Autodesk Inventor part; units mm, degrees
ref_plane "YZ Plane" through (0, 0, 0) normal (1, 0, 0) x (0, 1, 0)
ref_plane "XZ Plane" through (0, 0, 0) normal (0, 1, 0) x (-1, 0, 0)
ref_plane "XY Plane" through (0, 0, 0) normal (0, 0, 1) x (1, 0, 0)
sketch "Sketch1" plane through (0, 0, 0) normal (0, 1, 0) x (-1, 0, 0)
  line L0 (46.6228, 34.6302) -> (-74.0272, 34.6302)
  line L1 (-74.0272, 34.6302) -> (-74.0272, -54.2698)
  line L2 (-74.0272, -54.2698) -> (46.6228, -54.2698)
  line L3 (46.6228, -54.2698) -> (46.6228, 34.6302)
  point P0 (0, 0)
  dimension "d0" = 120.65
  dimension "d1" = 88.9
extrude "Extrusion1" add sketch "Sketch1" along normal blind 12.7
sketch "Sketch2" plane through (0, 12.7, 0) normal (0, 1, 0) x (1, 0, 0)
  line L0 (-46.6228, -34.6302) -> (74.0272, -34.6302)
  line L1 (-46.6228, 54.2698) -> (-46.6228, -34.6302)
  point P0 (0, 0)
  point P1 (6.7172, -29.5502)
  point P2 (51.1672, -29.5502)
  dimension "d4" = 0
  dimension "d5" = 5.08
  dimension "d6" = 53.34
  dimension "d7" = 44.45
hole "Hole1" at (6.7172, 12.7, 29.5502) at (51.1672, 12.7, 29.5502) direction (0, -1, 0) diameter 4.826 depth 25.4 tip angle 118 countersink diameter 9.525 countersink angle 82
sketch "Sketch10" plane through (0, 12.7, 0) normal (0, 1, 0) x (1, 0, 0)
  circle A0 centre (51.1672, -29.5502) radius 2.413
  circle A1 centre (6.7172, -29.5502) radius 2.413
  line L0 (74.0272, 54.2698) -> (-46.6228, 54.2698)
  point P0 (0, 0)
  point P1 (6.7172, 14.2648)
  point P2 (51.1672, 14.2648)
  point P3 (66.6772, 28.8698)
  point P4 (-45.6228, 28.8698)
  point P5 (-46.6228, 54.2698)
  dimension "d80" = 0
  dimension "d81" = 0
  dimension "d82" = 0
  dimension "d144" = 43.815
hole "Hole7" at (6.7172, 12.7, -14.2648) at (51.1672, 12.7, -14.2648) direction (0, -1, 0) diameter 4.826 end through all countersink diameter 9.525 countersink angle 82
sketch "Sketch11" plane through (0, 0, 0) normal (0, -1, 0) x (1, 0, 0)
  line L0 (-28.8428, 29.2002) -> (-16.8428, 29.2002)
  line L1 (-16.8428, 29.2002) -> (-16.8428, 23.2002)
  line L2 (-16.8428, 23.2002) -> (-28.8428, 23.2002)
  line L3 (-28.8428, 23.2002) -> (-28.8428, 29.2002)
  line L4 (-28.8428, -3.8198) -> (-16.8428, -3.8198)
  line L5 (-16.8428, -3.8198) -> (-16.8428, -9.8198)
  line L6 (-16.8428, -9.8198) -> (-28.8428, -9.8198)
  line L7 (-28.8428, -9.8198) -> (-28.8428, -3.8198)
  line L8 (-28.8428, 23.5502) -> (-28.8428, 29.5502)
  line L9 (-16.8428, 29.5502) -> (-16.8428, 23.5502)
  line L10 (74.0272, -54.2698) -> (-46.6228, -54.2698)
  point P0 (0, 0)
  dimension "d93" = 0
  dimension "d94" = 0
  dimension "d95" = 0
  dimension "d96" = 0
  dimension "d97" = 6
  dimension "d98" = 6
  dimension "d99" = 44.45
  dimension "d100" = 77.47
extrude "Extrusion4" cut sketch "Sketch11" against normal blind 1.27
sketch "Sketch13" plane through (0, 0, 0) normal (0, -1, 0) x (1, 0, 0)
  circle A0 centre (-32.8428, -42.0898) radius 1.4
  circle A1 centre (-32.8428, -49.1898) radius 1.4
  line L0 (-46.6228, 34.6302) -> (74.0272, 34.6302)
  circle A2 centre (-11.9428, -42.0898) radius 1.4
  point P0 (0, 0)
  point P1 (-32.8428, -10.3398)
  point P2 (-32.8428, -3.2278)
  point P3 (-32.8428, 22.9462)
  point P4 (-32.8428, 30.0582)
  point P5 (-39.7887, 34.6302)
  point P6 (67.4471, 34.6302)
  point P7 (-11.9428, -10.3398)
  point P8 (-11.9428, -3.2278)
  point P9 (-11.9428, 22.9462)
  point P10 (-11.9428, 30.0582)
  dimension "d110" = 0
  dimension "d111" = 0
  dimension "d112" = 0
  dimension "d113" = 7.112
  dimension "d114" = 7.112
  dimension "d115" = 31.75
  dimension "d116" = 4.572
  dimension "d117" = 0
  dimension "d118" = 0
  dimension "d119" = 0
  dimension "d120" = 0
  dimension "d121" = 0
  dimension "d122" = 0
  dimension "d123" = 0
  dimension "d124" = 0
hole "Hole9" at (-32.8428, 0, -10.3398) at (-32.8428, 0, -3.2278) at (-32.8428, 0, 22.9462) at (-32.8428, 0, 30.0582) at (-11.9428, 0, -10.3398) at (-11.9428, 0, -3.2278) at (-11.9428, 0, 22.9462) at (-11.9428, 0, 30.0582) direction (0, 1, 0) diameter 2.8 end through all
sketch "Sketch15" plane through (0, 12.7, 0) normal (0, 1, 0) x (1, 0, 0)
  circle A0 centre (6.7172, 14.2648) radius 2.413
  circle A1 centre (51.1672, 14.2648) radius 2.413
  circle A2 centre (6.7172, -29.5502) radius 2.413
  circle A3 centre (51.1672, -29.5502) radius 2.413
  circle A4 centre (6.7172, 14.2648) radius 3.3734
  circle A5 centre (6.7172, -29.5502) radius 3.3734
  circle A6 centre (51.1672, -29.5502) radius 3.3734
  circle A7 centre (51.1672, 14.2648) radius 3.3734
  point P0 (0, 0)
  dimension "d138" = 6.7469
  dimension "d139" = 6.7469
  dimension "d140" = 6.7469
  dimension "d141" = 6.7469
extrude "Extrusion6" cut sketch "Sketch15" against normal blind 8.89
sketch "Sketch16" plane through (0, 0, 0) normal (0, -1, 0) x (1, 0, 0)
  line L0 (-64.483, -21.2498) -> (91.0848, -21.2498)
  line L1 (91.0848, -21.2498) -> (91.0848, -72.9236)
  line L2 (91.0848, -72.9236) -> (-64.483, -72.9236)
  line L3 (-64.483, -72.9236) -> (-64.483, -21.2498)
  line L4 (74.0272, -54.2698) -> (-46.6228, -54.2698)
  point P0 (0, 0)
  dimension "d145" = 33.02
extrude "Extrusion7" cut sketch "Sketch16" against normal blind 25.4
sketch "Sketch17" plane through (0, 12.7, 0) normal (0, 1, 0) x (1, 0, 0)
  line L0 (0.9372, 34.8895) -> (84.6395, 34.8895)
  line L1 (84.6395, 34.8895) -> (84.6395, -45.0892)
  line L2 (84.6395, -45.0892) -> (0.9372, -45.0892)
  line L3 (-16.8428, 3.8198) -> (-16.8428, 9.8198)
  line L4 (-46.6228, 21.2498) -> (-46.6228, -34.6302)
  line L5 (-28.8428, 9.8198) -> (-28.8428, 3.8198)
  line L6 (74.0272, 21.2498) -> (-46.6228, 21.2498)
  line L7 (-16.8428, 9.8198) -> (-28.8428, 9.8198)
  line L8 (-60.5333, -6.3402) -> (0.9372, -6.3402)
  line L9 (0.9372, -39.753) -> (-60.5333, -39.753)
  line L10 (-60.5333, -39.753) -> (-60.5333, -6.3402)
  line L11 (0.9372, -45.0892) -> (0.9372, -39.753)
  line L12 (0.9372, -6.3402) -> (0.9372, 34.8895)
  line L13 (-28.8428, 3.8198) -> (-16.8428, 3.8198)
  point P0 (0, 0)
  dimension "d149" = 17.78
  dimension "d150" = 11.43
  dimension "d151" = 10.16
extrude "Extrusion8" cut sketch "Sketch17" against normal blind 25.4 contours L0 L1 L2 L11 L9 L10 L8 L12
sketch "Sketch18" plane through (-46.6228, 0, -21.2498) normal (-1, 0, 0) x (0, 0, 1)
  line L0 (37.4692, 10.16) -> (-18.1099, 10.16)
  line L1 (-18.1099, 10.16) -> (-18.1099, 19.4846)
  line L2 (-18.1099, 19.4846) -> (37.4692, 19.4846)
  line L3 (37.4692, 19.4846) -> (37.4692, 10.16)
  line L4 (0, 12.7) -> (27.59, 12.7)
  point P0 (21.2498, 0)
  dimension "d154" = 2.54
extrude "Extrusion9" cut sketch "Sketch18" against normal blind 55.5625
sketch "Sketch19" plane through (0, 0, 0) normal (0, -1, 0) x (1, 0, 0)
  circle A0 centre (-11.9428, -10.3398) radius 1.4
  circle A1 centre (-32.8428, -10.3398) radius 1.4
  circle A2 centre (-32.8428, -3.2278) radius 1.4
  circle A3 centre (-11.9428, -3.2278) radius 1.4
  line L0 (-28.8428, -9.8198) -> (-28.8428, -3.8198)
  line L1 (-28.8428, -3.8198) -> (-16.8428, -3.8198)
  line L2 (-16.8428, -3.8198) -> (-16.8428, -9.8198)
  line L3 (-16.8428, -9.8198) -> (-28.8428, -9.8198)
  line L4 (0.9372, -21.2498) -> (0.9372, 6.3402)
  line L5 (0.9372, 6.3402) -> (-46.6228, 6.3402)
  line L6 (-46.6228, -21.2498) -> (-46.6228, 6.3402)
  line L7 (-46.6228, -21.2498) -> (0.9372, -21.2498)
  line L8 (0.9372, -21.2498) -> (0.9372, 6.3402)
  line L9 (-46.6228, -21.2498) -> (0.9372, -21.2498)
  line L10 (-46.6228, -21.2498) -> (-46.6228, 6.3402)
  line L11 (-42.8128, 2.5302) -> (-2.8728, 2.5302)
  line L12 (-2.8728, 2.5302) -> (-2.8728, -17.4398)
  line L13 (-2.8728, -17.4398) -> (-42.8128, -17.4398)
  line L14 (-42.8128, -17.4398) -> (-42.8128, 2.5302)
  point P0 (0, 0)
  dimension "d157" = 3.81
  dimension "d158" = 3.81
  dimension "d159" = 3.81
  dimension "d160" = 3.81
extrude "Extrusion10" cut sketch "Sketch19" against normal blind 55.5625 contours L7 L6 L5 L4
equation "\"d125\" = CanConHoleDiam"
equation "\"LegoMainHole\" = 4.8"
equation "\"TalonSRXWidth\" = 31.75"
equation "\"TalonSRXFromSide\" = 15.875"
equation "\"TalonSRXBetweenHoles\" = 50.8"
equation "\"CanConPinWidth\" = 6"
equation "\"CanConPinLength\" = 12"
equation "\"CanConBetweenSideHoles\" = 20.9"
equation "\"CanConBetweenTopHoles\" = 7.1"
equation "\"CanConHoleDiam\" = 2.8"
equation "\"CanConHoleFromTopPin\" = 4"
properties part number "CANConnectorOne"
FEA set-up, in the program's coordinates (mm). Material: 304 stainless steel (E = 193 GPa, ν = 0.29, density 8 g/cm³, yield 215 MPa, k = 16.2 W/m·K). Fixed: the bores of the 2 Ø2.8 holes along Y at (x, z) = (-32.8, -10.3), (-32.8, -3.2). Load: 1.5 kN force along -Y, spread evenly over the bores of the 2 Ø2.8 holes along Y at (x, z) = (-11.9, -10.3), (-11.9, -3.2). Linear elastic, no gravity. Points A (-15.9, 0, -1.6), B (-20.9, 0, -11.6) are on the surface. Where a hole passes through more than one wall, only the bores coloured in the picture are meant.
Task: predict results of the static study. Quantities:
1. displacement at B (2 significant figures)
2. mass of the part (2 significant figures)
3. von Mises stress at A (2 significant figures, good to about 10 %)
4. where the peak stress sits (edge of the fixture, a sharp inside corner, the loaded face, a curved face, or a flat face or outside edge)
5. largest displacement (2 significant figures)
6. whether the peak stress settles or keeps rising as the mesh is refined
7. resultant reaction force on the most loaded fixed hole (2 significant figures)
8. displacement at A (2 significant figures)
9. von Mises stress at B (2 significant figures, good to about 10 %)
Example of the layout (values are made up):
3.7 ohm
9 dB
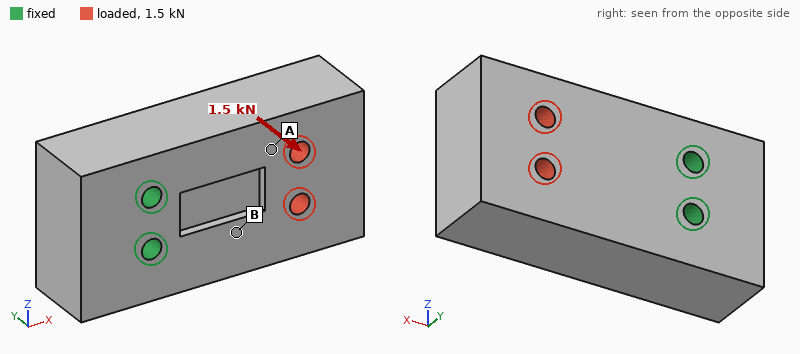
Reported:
9.0 µm
62 g
22 MPa
edge of the fixture
29 µm
keeps rising
760 N
14 µm
45 MPa
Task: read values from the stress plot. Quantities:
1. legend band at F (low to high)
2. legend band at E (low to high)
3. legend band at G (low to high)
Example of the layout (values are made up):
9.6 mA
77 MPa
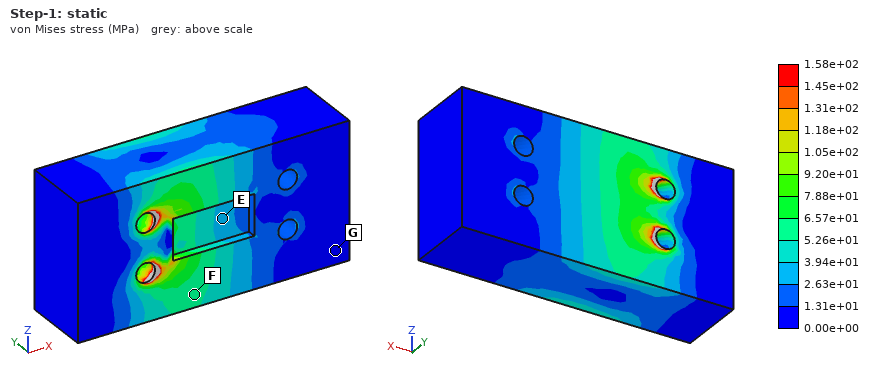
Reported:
5.26e+01 to 6.57e+01 MPa
2.63e+01 to 3.94e+01 MPa
0.00e+00 to 1.31e+01 MPa
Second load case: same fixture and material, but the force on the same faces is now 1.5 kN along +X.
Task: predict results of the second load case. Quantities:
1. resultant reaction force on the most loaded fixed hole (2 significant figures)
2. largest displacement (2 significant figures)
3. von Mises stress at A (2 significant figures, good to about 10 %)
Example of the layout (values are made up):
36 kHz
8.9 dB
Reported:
760 N
1.2 µm
9.6 MPa
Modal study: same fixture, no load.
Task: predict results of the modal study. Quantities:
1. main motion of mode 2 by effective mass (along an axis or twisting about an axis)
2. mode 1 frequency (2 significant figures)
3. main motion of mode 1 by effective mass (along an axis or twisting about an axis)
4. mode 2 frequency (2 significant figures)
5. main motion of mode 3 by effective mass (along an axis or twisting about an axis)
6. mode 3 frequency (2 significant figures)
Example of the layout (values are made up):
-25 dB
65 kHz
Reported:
along Z
8000 Hz
along Y
11 kHz
twisting about X
19 kHz
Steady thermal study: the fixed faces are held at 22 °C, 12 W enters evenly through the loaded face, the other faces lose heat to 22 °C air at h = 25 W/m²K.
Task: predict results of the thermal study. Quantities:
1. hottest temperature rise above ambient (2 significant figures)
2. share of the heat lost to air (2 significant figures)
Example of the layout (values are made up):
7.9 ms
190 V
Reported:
74 K
19 %
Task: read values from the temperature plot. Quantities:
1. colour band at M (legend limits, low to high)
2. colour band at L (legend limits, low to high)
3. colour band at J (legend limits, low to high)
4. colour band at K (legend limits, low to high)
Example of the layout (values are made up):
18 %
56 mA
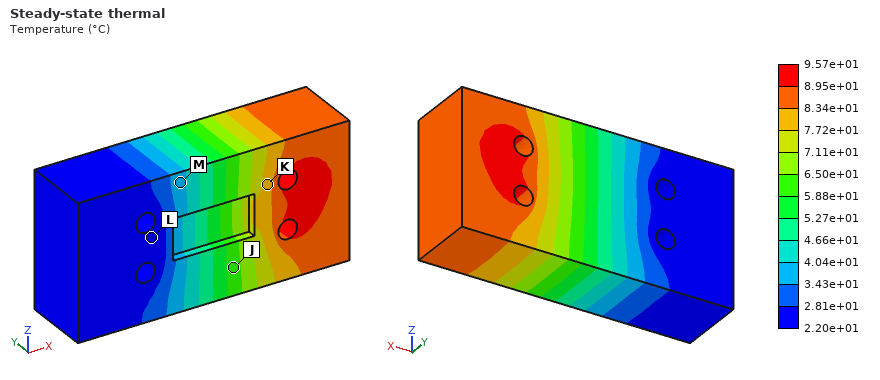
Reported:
3.43e+01 to 4.04e+01 °C
2.20e+01 to 2.81e+01 °C
5.88e+01 to 6.50e+01 °C
7.72e+01 to 8.34e+01 °C
